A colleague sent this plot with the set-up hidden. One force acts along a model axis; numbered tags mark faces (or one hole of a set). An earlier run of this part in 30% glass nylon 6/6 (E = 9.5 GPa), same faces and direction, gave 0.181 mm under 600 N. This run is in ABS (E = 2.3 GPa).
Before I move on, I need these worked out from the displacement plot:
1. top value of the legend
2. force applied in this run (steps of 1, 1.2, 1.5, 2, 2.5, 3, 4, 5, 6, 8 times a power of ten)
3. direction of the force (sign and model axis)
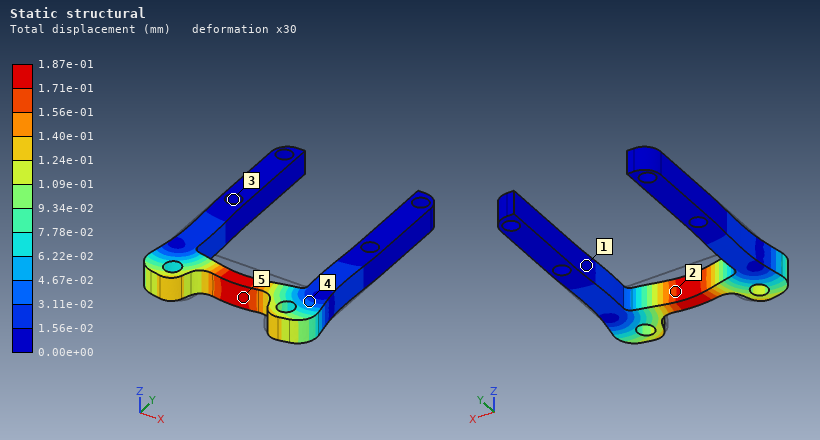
1.87e-01 mm
150 N
-Y
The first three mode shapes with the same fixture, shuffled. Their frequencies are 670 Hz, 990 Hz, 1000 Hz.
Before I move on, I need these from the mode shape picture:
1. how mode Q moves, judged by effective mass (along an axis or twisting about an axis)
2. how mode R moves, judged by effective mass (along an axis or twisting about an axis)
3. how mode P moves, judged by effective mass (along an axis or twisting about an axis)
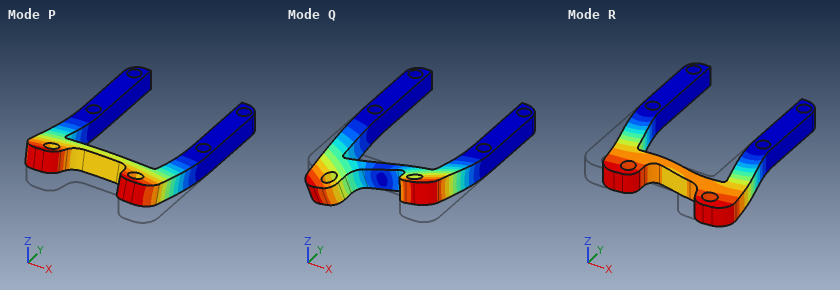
twisting about Y
along X
along Z
